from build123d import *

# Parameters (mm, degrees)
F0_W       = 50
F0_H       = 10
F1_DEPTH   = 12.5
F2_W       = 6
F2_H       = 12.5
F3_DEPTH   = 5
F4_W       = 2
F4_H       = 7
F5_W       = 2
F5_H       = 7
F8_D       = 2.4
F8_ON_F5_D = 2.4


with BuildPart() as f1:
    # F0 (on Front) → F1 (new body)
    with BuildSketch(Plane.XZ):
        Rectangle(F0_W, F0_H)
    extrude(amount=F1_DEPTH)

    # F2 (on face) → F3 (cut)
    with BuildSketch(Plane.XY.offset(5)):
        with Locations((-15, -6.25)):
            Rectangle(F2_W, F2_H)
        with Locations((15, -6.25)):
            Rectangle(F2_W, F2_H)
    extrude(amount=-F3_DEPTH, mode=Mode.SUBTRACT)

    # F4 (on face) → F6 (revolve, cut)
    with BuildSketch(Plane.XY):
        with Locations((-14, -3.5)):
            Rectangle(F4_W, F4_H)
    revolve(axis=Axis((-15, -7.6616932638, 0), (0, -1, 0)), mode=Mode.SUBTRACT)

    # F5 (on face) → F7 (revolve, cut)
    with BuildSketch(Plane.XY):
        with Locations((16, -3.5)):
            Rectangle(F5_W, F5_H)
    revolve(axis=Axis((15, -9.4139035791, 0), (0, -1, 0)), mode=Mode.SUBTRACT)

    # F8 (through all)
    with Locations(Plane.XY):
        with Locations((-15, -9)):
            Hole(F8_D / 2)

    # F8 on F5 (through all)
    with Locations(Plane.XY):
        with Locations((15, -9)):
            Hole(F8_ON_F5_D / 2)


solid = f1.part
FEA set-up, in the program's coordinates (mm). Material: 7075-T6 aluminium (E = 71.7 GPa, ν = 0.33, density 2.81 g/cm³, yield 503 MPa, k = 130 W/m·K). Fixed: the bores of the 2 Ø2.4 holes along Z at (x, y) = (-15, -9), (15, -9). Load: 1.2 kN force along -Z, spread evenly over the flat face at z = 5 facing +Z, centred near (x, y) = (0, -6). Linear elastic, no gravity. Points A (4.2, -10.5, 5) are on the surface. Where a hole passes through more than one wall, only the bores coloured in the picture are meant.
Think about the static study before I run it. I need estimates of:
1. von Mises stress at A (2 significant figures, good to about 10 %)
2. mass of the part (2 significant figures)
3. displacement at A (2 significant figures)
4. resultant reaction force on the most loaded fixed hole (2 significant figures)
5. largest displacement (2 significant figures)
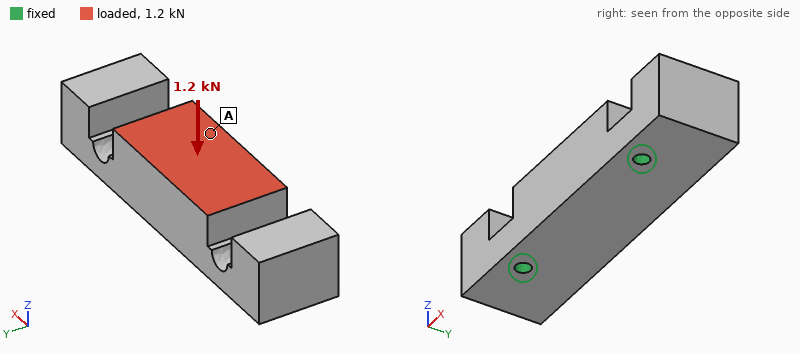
14 MPa
15 g
8.3 µm
660 N
16 µm
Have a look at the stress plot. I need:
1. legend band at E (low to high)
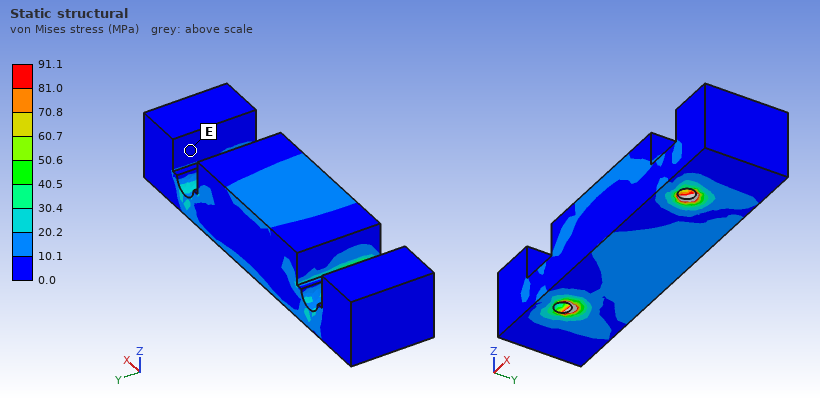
0.0 to 10.1 MPa
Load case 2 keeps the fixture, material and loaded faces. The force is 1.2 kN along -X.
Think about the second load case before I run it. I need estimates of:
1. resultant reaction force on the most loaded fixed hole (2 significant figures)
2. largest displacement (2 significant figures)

690 N
4.5 µm
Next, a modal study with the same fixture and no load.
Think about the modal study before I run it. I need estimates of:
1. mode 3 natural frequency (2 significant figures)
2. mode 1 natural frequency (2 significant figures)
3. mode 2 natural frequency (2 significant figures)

17 kHz
14 kHz
16 kHz
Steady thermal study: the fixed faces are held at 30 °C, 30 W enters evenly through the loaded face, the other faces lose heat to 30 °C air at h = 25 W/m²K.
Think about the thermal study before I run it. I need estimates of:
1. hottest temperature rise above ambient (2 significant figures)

20 K
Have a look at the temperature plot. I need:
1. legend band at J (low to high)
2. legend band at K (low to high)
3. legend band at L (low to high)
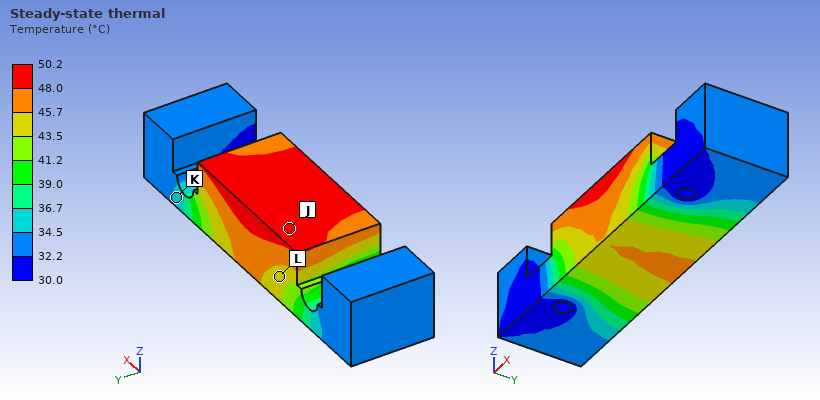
48.0 to 50.2 °C
34.5 to 36.7 °C
43.5 to 45.7 °C
